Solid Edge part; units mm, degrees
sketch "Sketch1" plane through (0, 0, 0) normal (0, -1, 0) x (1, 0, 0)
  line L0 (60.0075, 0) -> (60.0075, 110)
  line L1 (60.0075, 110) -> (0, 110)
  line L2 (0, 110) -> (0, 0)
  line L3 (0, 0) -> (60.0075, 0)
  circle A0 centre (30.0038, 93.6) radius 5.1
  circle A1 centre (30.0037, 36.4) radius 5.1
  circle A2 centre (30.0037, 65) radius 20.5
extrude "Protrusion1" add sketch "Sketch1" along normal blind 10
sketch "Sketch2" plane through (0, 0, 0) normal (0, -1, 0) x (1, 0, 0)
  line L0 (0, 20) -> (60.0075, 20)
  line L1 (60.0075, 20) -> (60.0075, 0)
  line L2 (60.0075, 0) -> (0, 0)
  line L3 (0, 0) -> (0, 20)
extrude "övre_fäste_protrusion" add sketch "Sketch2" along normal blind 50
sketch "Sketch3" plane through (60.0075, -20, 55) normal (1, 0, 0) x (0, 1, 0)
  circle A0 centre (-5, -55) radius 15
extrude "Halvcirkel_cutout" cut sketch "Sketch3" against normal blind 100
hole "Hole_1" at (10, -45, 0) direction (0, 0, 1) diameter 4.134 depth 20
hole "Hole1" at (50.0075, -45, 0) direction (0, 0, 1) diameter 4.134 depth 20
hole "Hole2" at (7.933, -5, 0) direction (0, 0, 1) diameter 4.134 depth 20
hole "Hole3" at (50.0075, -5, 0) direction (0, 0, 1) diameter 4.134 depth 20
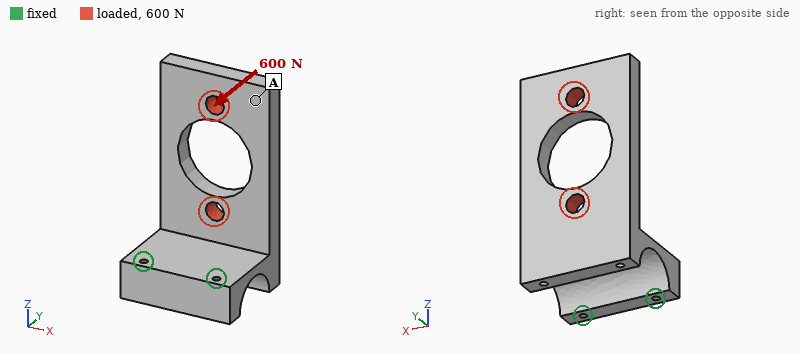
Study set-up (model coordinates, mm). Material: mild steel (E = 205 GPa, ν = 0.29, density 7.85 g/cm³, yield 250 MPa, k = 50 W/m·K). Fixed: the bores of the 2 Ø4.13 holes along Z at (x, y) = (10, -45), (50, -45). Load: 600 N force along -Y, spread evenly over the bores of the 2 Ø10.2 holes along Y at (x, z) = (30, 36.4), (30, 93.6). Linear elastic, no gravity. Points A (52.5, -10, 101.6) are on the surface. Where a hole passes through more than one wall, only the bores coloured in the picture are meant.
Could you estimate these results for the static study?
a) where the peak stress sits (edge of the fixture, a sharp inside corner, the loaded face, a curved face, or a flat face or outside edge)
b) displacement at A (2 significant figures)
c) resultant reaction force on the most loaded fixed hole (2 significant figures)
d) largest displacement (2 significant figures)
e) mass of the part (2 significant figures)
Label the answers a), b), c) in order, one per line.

a) a flat face or outside edge
b) 0.37 mm
c) 300 N
d) 0.42 mm
e) 600 g
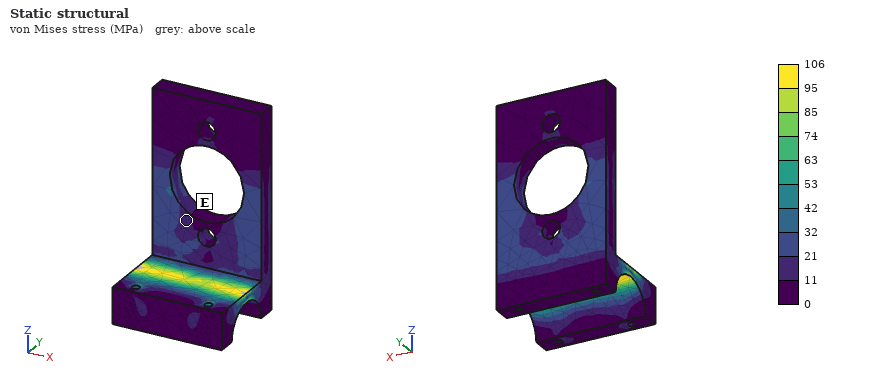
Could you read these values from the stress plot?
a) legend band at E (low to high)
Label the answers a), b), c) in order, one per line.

a) 11 to 21 MPa
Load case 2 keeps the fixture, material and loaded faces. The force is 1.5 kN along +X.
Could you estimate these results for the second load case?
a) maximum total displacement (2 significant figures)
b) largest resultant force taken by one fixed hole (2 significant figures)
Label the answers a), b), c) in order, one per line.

a) 0.16 mm
b) 2.3 kN
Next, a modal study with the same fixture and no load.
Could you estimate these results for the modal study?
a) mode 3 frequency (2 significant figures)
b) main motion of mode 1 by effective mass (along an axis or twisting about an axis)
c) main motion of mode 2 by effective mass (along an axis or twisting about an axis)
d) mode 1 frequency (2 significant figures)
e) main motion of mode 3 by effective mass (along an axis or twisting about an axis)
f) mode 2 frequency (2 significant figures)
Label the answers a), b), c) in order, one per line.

a) 1800 Hz
b) along Y
c) along X
d) 390 Hz
e) along Z
f) 1000 Hz
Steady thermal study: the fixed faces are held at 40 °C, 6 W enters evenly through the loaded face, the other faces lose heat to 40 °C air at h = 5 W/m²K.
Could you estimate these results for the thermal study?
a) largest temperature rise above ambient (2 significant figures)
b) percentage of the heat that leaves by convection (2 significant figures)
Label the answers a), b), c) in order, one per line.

a) 24 K
b) 20 %
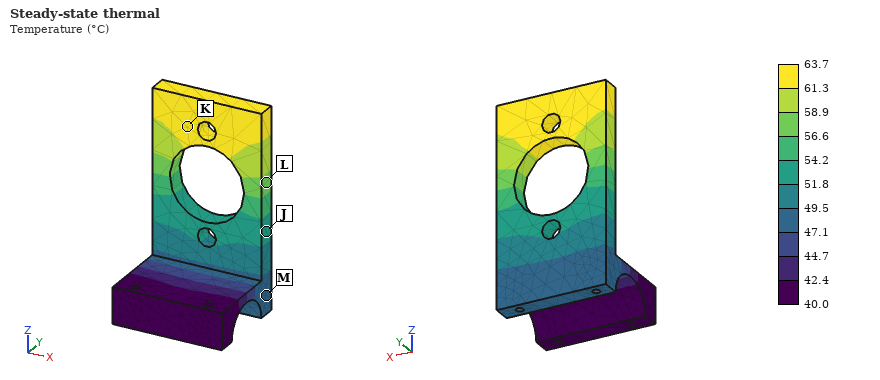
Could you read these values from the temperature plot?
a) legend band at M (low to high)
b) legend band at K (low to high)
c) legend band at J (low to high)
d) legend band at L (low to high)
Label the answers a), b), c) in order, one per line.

a) 47.1 to 49.5 °C
b) 61.3 to 63.7 °C
c) 51.8 to 54.2 °C
d) 56.6 to 58.9 °C
